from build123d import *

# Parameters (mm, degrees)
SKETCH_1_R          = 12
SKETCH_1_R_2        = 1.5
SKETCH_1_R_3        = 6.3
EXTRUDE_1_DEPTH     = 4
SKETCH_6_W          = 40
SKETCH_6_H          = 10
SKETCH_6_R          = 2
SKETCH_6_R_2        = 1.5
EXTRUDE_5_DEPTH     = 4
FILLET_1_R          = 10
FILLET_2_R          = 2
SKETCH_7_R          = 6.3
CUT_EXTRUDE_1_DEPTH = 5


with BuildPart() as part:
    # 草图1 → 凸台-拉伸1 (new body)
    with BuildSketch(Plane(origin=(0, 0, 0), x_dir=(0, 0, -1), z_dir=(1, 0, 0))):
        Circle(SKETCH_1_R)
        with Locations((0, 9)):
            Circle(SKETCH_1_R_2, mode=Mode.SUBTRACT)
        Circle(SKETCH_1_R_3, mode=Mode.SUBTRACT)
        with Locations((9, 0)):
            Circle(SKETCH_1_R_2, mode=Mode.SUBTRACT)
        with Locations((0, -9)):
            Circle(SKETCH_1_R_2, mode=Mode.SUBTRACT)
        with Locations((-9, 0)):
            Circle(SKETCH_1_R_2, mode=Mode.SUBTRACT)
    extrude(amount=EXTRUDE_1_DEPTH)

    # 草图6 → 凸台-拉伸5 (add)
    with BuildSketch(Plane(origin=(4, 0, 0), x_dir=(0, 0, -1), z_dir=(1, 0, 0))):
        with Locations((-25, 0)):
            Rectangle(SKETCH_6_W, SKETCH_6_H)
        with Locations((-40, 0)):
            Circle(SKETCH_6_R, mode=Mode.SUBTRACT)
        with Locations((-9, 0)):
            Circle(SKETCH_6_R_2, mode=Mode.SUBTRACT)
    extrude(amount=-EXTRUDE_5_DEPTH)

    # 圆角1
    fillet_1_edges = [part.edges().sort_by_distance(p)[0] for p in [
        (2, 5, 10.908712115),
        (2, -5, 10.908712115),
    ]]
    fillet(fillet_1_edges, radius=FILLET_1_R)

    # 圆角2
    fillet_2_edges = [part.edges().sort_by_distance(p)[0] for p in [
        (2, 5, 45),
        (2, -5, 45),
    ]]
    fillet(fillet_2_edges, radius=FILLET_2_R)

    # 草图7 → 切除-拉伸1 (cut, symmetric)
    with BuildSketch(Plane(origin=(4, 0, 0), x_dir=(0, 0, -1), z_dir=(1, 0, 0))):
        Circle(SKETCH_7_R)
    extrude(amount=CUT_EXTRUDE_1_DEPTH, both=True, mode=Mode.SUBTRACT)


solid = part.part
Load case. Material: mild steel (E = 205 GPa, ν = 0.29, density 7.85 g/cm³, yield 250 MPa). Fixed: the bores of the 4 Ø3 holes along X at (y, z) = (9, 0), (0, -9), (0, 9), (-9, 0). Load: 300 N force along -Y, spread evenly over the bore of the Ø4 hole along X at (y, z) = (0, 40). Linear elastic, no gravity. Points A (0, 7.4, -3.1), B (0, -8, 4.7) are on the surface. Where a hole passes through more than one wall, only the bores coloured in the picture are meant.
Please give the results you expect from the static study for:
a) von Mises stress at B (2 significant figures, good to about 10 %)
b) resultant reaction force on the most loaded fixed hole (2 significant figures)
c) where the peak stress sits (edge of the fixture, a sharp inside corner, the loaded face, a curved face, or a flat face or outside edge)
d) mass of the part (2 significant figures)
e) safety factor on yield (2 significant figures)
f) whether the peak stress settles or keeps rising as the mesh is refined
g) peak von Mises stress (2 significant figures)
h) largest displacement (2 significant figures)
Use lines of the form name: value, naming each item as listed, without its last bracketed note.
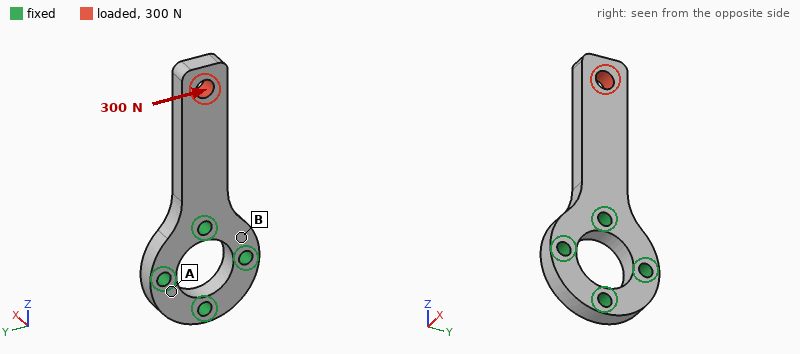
von Mises stress at B: 30 MPa
resultant reaction force on the most loaded fixed hole: 500 N
where the peak stress sits: a curved face
mass of the part: 20 g
safety factor on yield: 2.0
whether the peak stress settles or keeps rising as the mesh is refined: settles
peak von Mises stress: 130 MPa
largest displacement: 57 µm
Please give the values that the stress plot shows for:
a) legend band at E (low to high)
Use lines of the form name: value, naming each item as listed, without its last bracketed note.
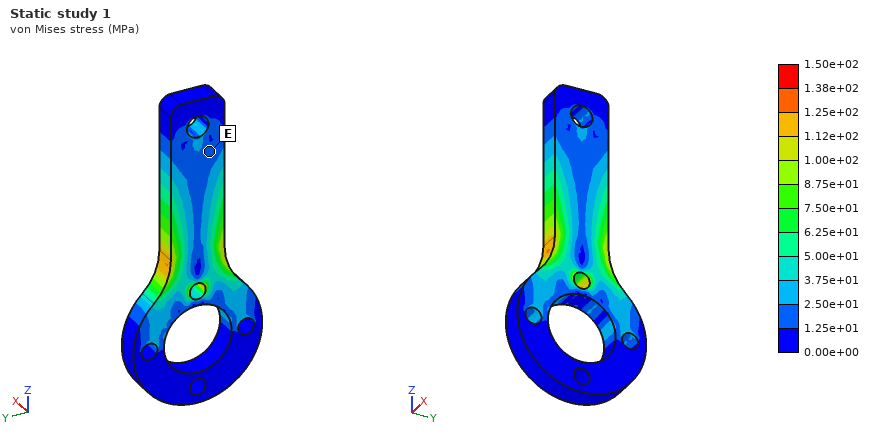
legend band at E: 1.25e+01 to 2.50e+01 MPa
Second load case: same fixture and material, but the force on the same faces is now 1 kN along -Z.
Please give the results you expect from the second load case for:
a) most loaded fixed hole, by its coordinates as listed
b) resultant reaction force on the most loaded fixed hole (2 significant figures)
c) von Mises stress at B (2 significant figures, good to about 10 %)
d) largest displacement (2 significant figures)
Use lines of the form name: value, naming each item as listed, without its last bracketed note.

most loaded fixed hole, by its coordinates as listed: (0, 9)
resultant reaction force on the most loaded fixed hole: 780 N
von Mises stress at B: 6.5 MPa
largest displacement: 4.7 µm
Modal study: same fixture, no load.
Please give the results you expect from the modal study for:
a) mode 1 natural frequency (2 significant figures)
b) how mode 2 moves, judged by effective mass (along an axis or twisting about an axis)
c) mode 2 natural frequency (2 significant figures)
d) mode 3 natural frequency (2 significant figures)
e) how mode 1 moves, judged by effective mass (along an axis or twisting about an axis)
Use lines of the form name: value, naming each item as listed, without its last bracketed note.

mode 1 natural frequency: 2800 Hz
how mode 2 moves, judged by effective mass: along Y
mode 2 natural frequency: 6500 Hz
mode 3 natural frequency: 15 kHz
how mode 1 moves, judged by effective mass: along X
